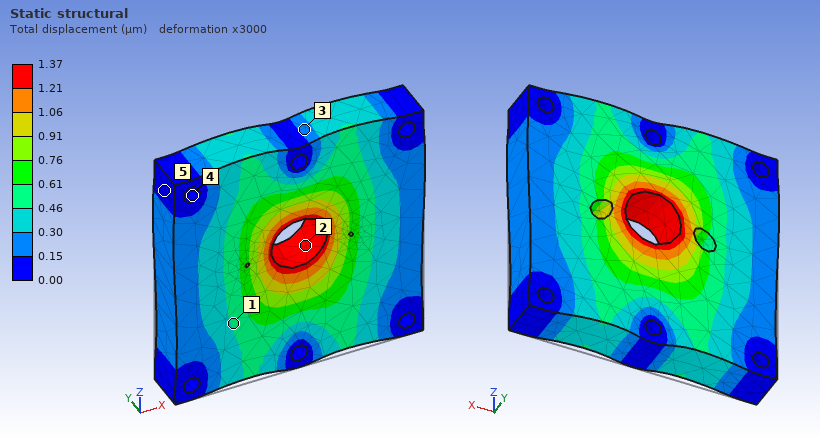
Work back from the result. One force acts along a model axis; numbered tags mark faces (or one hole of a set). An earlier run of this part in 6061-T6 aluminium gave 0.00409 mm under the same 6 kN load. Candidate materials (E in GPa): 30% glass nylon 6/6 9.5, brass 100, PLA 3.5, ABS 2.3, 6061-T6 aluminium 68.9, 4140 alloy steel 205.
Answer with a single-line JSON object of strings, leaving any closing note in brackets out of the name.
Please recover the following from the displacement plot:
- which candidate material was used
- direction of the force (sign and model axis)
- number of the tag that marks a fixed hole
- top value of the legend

{"which candidate material was used": "4140 alloy steel", "direction of the force": "+Z", "number of the tag that marks a fixed hole": "4", "top value of the legend": "1.37 µm"}
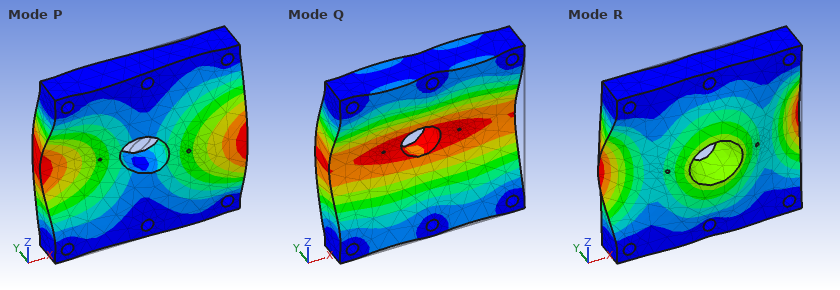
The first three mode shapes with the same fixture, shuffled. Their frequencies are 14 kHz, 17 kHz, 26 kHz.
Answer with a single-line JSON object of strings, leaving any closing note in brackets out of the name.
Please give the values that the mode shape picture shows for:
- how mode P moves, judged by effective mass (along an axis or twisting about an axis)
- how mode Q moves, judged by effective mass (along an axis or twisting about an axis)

{"how mode P moves, judged by effective mass": "twisting about Z", "how mode Q moves, judged by effective mass": "along Y"}
